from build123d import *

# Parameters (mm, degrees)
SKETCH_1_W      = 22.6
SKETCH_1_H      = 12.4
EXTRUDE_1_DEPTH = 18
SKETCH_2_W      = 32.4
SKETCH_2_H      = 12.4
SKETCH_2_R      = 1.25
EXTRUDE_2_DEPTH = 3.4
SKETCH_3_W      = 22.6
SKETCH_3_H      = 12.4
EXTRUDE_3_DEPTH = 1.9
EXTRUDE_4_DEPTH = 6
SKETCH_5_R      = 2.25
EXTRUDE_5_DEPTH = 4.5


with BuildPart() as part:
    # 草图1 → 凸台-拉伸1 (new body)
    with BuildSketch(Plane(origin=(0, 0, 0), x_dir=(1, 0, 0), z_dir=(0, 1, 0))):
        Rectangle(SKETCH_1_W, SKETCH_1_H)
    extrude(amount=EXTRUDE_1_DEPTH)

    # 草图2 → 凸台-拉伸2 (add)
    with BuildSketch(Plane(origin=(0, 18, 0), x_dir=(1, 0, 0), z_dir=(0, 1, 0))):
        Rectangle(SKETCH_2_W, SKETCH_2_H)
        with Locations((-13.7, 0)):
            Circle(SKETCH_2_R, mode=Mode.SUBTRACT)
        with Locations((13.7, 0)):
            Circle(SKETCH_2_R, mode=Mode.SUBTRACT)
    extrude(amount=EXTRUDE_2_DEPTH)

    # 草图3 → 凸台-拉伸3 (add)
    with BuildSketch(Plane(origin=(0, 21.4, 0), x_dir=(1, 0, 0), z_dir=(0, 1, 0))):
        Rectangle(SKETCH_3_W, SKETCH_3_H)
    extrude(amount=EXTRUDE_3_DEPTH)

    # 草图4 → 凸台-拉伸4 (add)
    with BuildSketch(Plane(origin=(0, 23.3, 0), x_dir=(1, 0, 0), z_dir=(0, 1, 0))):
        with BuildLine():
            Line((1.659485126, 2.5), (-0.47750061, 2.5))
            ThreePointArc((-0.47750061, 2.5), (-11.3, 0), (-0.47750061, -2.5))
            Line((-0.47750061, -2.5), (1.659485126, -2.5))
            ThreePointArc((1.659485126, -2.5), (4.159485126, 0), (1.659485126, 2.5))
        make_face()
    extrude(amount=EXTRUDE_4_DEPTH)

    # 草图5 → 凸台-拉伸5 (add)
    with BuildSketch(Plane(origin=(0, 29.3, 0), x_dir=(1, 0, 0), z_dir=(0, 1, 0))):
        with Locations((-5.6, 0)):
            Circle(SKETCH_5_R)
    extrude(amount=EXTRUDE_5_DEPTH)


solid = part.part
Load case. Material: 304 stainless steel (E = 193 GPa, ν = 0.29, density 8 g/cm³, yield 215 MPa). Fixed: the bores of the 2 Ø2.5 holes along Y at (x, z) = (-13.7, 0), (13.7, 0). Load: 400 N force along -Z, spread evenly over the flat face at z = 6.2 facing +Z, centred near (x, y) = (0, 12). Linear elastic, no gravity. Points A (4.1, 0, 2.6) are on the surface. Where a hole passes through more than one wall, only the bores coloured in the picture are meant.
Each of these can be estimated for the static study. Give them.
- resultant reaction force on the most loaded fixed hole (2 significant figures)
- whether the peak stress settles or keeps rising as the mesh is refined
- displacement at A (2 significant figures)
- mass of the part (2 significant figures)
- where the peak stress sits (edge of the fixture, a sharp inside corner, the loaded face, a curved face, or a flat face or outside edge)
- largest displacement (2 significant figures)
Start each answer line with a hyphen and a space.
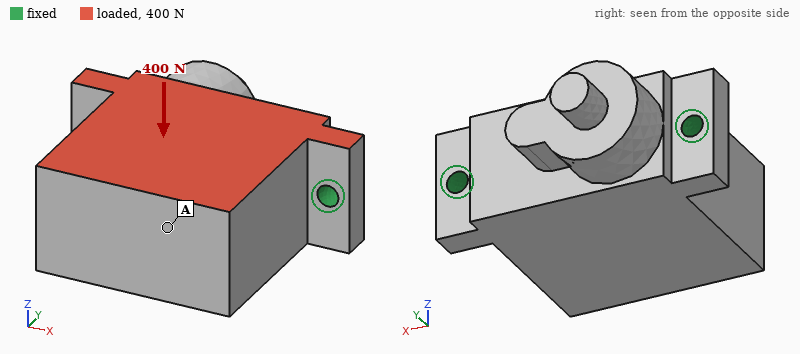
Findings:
- 200 N
- keeps rising
- 10 µm
- 62 g
- edge of the fixture
- 11 µm
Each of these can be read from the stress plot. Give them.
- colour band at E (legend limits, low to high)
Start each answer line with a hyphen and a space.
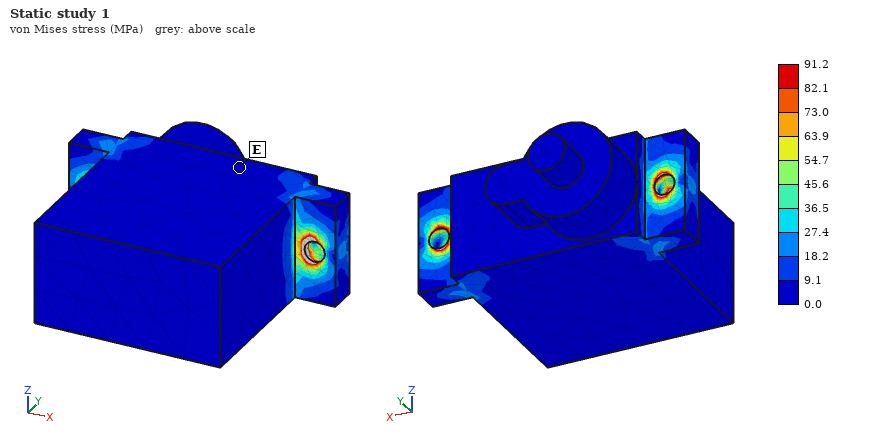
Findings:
- 0.0 to 9.1 MPa
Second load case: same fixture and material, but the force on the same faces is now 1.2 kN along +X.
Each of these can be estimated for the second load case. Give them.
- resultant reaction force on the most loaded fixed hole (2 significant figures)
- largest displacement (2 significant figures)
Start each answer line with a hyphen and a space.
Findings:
- 760 N
- 3.6 µm
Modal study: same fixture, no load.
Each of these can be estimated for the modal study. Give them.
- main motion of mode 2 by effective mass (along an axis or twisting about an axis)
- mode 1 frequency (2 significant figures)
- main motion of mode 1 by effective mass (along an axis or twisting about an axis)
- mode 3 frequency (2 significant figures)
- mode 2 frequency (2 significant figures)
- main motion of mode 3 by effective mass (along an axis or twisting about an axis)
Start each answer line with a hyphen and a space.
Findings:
- along X
- 4700 Hz
- along Z
- 18 kHz
- 17 kHz
- along Y
